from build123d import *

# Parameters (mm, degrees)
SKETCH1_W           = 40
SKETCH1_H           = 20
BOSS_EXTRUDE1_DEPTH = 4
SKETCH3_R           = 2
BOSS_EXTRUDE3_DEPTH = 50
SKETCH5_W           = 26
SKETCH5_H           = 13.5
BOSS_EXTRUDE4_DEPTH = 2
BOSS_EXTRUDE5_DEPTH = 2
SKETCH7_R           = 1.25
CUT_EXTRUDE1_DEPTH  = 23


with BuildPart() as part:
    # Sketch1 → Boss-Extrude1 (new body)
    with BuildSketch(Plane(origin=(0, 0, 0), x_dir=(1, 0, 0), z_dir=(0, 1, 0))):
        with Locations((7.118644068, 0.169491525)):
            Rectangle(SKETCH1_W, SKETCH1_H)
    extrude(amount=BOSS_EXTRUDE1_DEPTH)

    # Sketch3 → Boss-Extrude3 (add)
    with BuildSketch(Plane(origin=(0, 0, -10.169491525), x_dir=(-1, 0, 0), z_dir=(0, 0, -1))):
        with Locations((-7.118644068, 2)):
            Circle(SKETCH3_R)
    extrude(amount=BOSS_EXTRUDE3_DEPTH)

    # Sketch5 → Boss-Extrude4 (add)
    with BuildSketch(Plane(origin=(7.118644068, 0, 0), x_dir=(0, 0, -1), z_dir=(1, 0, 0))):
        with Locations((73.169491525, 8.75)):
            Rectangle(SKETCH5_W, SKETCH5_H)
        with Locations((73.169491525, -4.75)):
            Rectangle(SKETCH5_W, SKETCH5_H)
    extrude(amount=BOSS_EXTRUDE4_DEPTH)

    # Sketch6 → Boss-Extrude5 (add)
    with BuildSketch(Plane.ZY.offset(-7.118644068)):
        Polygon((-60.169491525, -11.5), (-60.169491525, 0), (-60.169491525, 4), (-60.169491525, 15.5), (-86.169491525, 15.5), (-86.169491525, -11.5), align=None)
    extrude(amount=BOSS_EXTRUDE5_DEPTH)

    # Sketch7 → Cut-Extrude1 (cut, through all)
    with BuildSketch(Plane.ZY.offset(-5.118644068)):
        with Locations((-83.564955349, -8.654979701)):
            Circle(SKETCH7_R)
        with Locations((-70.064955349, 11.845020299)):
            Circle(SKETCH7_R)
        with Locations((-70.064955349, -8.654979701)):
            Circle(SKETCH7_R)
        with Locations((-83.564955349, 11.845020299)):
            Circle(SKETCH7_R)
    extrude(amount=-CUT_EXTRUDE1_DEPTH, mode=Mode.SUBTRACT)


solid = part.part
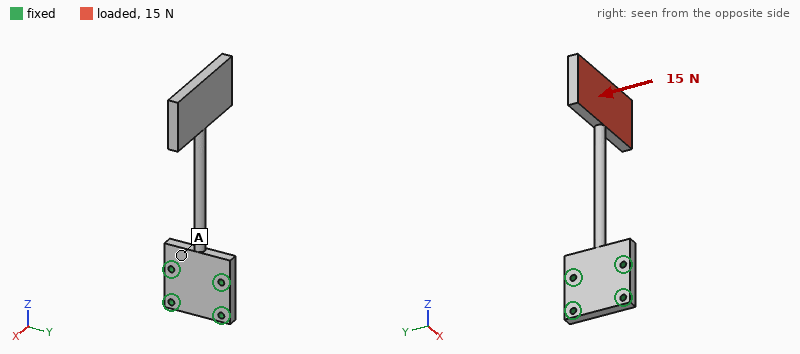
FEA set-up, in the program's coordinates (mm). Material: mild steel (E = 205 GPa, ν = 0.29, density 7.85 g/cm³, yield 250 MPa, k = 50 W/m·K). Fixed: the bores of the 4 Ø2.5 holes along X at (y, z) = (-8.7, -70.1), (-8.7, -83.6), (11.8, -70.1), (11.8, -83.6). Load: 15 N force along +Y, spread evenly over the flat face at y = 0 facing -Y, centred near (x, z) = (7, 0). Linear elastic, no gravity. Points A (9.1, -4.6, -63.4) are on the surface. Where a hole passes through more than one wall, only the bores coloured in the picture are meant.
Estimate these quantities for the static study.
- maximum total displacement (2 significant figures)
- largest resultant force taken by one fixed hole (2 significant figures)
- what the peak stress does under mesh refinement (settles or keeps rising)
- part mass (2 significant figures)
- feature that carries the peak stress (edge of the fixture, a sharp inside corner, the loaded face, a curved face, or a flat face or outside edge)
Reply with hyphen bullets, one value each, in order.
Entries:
- 0.55 mm
- 47 N
- keeps rising
- 51 g
- a sharp inside corner
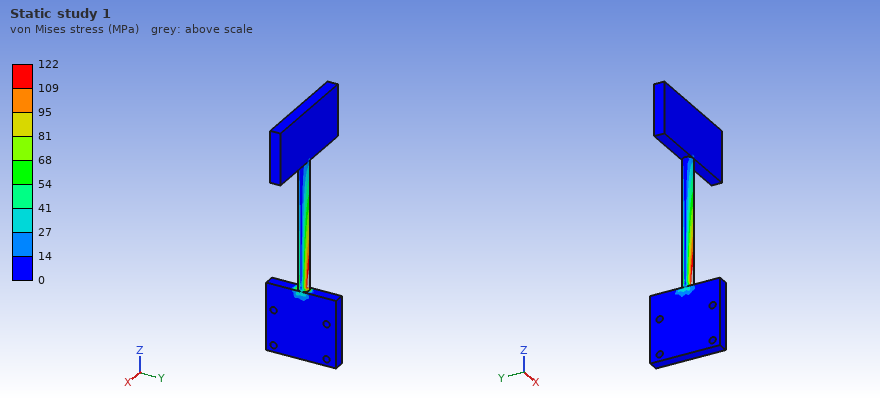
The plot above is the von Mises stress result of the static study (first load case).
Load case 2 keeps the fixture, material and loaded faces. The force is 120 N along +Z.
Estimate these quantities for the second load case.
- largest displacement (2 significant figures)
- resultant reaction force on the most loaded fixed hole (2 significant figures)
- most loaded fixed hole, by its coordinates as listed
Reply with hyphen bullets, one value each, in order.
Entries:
- 0.22 mm
- 54 N
- (-8.7, -70.1)
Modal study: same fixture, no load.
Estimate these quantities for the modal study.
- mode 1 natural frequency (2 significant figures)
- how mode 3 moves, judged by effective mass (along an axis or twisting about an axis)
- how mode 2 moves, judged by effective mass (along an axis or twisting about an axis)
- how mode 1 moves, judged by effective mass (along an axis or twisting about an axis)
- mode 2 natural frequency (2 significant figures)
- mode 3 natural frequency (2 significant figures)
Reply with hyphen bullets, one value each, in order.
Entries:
- 170 Hz
- twisting about Z
- along Y
- along X
- 180 Hz
- 530 Hz
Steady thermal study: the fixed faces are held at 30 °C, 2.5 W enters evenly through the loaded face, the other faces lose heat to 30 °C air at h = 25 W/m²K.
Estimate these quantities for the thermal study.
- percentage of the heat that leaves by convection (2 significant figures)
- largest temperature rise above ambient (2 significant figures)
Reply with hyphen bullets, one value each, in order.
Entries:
- 82 %
- 53 K
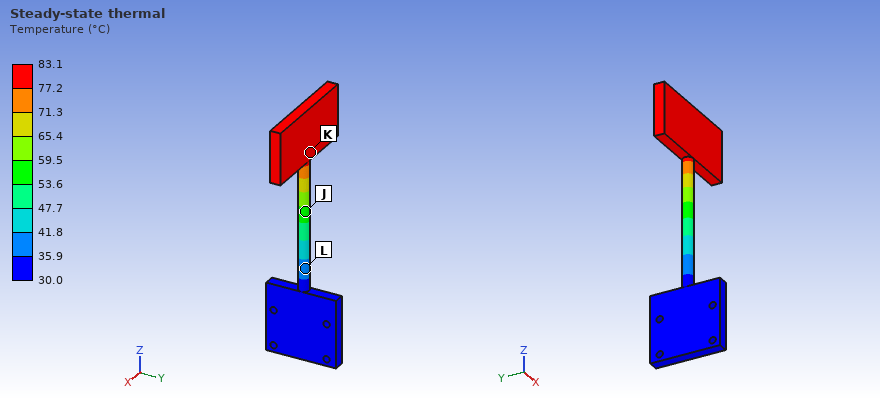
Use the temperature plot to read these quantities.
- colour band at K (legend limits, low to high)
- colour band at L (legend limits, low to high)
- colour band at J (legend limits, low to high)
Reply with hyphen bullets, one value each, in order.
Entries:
- 77.2 to 83.1 °C
- 35.9 to 41.8 °C
- 53.6 to 59.5 °C
